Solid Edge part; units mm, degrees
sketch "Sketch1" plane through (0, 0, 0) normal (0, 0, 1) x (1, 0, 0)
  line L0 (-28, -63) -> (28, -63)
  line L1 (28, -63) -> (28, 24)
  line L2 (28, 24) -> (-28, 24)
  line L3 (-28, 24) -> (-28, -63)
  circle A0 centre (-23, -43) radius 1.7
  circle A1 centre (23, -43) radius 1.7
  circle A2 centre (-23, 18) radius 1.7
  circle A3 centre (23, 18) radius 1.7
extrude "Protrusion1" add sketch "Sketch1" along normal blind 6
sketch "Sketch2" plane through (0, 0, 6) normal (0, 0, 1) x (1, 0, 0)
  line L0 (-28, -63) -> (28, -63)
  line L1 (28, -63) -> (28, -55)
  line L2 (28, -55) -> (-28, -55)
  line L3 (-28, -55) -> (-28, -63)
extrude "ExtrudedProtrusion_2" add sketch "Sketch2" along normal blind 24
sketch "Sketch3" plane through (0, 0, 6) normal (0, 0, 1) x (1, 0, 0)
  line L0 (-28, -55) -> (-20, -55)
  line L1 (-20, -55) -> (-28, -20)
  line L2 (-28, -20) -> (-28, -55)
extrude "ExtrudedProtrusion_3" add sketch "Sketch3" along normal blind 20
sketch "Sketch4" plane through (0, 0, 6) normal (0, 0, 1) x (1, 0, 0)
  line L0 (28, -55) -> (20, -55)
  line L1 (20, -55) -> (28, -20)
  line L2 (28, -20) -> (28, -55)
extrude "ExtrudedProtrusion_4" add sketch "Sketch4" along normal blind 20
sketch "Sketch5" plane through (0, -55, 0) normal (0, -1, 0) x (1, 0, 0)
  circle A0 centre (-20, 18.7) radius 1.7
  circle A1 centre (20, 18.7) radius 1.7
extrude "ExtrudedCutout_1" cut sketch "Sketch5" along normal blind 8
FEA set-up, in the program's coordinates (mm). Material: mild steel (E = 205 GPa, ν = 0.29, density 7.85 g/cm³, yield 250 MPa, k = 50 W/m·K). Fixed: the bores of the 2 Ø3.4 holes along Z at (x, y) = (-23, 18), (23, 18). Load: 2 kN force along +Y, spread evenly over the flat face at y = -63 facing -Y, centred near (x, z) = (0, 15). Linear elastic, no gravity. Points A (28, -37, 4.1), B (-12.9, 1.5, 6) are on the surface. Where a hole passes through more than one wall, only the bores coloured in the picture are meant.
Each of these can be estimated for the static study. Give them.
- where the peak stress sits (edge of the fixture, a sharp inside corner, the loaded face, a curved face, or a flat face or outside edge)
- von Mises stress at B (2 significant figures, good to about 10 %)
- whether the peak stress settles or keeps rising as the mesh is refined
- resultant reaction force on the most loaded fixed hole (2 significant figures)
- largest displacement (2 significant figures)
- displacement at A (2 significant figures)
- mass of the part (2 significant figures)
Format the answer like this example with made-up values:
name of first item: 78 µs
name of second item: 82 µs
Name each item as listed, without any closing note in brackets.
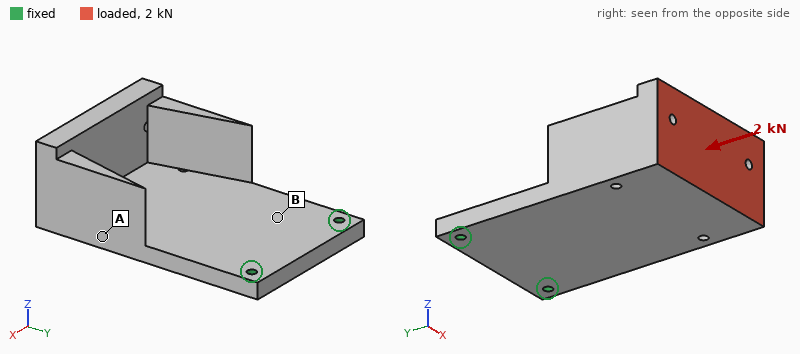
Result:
where the peak stress sits: edge of the fixture
von Mises stress at B: 75 MPa
whether the peak stress settles or keeps rising as the mesh is refined: keeps rising
resultant reaction force on the most loaded fixed hole: 1.0 kN
largest displacement: 0.44 mm
displacement at A: 0.22 mm
mass of the part: 350 g
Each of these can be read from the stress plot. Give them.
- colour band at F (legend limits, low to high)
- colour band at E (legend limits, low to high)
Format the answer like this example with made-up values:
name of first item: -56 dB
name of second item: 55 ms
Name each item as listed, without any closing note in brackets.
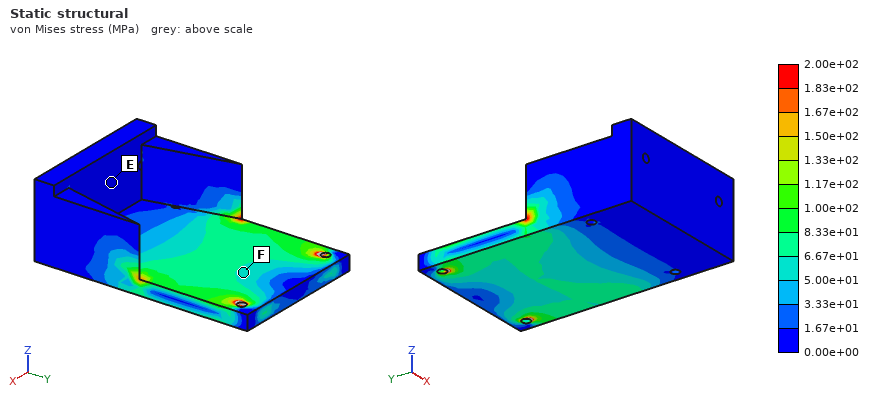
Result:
colour band at F: 5.00e+01 to 6.67e+01 MPa
colour band at E: 0.00e+00 to 1.67e+01 MPa
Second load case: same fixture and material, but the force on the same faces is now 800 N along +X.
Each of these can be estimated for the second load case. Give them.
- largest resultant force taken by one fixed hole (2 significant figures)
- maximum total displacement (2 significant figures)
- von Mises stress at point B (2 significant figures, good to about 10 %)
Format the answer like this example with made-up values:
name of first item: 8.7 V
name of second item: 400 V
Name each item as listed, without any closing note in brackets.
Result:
largest resultant force taken by one fixed hole: 1.5 kN
maximum total displacement: 50 µm
von Mises stress at point B: 23 MPa
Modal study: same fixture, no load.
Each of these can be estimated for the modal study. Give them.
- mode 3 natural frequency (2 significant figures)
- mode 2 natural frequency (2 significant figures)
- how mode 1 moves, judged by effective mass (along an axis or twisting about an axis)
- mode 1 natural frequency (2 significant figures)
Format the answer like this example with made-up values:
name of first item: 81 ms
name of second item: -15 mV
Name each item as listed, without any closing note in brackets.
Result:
mode 3 natural frequency: 3000 Hz
mode 2 natural frequency: 1400 Hz
how mode 1 moves, judged by effective mass: along Z
mode 1 natural frequency: 390 Hz
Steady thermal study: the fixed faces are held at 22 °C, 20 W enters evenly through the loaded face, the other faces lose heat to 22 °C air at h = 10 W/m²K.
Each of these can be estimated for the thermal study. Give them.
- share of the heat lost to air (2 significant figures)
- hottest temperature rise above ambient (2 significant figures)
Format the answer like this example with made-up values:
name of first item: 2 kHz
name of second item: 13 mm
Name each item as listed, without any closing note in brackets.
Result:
share of the heat lost to air: 34 %
hottest temperature rise above ambient: 72 K
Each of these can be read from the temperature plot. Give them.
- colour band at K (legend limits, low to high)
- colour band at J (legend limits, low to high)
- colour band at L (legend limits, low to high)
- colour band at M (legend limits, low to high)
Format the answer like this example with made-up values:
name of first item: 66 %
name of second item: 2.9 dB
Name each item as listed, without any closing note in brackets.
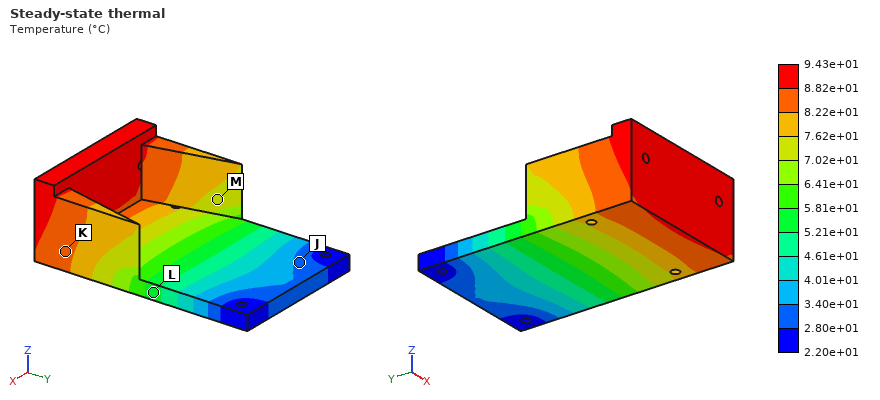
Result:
colour band at K: 8.22e+01 to 8.82e+01 °C
colour band at J: 2.80e+01 to 3.40e+01 °C
colour band at L: 5.21e+01 to 5.81e+01 °C
colour band at M: 7.02e+01 to 7.62e+01 °C
